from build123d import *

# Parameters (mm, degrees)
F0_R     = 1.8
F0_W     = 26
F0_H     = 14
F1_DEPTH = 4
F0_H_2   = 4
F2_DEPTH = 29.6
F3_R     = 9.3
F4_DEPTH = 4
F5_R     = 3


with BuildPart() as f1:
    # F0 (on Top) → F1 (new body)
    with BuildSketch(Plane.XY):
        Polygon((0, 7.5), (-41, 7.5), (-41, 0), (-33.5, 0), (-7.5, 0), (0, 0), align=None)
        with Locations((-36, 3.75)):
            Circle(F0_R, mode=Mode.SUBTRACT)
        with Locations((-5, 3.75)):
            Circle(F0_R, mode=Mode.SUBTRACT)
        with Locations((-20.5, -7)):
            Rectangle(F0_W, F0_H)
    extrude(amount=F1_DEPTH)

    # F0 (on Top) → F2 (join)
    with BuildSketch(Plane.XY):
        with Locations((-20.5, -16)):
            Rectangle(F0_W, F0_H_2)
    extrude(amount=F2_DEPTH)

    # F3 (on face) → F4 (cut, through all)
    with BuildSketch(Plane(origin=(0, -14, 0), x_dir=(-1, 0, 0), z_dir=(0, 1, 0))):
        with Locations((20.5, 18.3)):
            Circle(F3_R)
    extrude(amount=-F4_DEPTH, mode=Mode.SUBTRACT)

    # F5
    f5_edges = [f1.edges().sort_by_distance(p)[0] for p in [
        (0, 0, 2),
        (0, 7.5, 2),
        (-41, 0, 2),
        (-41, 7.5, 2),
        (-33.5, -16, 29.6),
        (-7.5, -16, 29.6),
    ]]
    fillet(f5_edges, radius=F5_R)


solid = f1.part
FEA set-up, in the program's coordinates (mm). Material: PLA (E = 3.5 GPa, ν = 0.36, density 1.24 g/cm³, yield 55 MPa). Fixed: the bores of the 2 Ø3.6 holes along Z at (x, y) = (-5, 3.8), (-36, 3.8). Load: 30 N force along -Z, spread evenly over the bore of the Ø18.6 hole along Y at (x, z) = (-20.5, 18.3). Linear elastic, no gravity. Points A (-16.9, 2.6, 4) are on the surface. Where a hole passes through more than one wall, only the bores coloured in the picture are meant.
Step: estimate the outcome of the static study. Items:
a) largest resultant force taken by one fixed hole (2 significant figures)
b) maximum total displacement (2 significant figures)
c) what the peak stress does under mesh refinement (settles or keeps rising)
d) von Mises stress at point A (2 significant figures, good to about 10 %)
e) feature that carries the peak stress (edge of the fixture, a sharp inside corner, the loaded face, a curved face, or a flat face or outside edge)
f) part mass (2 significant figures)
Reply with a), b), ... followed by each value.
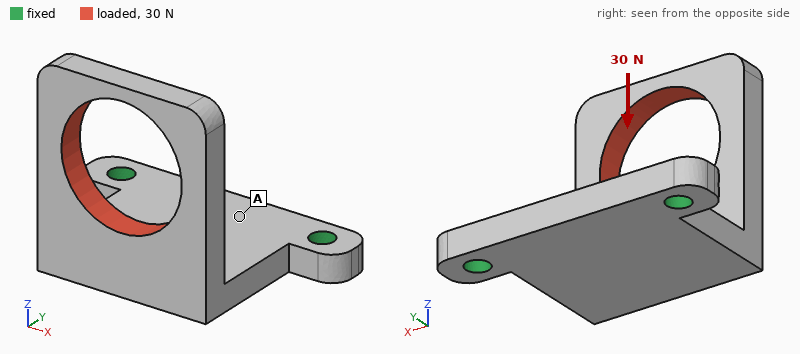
a) 15 N
b) 0.61 mm
c) keeps rising
d) 3.2 MPa
e) edge of the fixture
f) 5.6 g
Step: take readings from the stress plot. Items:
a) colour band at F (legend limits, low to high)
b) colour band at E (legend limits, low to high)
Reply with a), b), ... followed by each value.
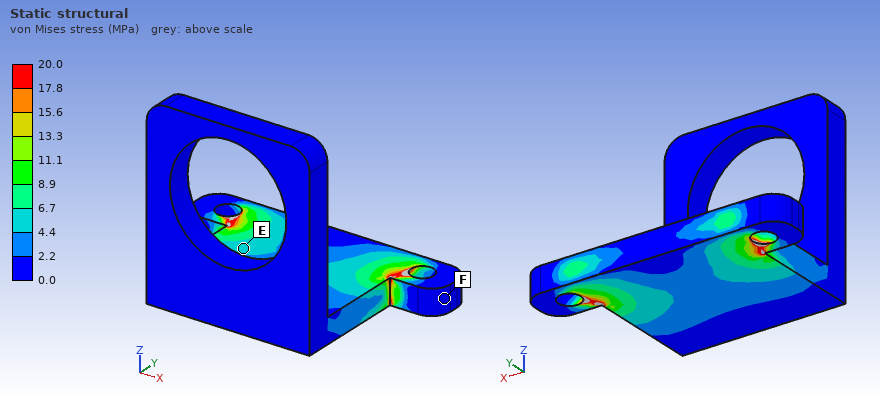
a) 0.0 to 2.2 MPa
b) 4.4 to 6.7 MPa
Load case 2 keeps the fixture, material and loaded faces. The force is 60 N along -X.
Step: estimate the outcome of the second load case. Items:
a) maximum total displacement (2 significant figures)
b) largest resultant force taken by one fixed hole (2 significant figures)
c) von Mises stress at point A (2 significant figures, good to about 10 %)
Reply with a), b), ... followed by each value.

a) 0.63 mm
b) 66 N
c) 4.5 MPa
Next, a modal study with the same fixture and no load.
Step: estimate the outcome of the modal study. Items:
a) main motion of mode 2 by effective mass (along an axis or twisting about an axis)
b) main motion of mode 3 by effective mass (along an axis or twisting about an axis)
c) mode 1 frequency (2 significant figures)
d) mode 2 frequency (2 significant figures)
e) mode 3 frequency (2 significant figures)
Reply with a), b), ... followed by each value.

a) along X
b) along Z
c) 670 Hz
d) 1300 Hz
e) 1600 Hz
